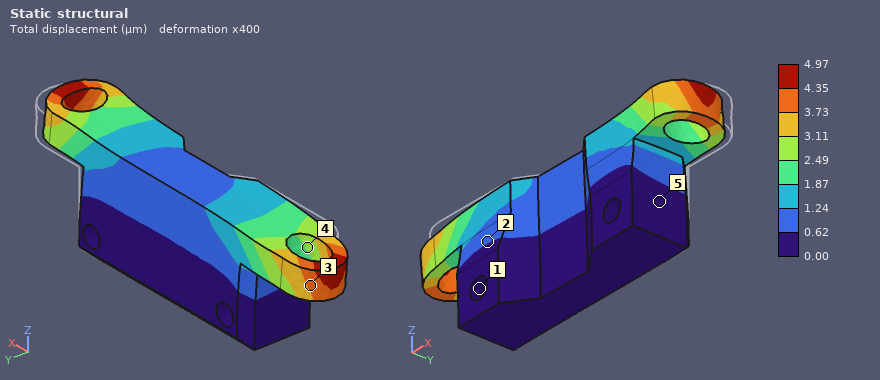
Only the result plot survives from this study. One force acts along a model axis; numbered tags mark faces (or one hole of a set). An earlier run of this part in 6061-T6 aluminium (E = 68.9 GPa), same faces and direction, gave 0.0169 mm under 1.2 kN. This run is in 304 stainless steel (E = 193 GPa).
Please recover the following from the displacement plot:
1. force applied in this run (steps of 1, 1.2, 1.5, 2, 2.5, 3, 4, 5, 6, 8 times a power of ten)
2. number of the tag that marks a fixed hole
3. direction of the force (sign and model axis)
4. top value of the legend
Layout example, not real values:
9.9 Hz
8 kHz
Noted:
1 kN
1
-X
4.97 µm
